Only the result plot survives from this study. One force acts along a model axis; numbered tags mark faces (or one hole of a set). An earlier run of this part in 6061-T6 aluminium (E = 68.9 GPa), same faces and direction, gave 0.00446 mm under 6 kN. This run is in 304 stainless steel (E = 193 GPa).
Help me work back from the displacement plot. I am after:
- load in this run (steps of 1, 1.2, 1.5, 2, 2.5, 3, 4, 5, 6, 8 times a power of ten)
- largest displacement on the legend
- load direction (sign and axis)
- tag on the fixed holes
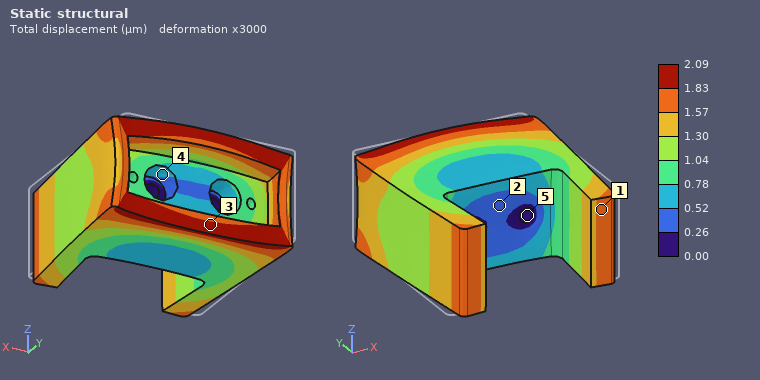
8 kN
2.09 µm
-Y
5
